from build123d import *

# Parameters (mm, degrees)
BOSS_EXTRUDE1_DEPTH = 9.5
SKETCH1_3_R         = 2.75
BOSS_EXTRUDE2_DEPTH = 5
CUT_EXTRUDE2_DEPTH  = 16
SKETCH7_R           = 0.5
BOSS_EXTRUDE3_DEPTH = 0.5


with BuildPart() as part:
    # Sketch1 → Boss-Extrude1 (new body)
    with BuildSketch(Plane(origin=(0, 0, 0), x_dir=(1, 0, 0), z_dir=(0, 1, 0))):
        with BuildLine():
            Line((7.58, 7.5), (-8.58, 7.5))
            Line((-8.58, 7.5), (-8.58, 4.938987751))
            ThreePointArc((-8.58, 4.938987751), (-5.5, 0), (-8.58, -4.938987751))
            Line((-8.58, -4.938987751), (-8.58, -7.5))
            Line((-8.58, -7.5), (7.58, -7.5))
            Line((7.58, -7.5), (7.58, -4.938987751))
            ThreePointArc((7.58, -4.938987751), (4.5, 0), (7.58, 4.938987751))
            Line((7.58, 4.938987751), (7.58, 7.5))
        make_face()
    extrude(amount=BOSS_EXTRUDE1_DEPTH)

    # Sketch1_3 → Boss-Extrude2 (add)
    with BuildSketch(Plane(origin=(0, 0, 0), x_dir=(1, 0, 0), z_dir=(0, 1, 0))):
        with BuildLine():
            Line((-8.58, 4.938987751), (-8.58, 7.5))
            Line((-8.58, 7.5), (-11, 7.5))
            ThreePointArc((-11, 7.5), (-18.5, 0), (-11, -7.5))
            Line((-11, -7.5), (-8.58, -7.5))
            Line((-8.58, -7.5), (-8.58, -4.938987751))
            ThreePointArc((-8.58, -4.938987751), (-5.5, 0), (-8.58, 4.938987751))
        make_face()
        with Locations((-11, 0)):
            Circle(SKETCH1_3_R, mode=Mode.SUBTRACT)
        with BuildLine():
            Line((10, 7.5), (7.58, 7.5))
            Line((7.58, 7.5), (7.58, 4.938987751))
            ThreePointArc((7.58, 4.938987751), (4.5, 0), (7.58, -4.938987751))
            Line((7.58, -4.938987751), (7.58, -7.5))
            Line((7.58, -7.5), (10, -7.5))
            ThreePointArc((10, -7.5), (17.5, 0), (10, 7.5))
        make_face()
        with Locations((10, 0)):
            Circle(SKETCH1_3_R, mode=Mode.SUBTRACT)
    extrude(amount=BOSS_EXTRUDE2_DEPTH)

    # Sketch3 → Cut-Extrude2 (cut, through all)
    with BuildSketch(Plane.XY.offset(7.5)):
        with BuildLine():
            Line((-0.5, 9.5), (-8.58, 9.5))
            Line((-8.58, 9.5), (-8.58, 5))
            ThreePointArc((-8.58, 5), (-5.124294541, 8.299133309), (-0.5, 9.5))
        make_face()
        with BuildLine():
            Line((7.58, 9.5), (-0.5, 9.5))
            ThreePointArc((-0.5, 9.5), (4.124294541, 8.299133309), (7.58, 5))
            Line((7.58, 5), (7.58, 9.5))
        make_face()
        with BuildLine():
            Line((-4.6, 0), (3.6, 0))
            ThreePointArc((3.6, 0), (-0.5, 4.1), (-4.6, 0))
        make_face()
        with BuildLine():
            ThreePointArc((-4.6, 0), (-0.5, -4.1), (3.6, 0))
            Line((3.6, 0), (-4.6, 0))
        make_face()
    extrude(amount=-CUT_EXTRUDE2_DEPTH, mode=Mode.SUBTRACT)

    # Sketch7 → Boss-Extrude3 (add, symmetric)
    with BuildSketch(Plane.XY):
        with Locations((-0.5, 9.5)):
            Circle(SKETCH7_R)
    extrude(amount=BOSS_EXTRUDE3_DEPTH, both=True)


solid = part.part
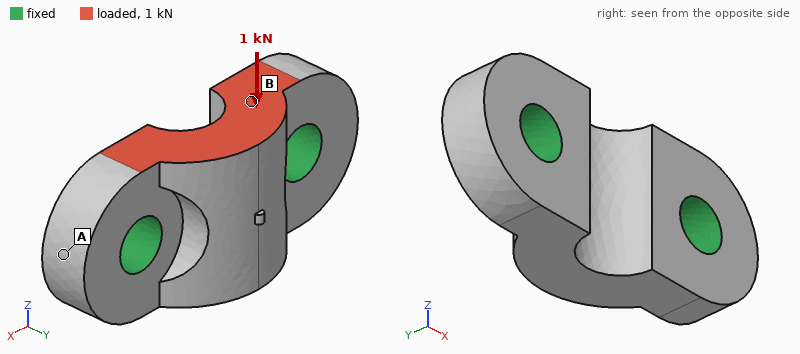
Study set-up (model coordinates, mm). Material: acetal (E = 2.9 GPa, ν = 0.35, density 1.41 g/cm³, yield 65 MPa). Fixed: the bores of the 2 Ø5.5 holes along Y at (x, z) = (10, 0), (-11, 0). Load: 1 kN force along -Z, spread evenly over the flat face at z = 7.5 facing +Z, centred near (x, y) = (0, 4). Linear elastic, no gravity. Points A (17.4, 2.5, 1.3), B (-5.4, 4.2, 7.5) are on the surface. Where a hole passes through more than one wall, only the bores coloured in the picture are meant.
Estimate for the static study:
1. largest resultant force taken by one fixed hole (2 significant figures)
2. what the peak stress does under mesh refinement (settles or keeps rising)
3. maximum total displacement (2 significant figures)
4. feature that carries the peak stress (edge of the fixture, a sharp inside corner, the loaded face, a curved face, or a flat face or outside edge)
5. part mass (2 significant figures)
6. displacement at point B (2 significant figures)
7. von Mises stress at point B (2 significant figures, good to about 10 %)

500 N
keeps rising
0.13 mm
edge of the fixture
3.6 g
0.076 mm
13 MPa
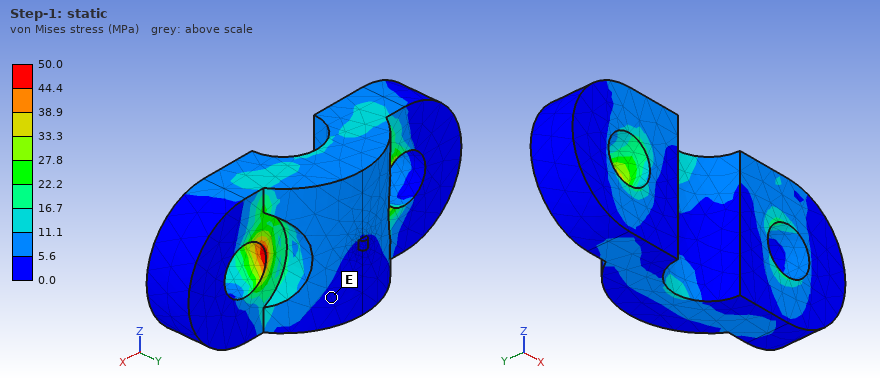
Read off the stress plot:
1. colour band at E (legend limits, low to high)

0.0 to 5.6 MPa
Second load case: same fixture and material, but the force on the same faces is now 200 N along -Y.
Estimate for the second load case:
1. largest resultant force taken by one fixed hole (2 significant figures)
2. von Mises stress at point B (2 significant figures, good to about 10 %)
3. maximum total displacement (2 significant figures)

110 N
3.8 MPa
62 µm
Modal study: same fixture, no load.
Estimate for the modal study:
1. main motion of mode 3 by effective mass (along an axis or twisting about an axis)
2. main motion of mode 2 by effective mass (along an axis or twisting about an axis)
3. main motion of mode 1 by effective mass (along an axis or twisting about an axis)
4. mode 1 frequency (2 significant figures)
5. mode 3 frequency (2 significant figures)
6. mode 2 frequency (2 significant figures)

along Z
along Y
along Z
10 kHz
20 kHz
15 kHz
